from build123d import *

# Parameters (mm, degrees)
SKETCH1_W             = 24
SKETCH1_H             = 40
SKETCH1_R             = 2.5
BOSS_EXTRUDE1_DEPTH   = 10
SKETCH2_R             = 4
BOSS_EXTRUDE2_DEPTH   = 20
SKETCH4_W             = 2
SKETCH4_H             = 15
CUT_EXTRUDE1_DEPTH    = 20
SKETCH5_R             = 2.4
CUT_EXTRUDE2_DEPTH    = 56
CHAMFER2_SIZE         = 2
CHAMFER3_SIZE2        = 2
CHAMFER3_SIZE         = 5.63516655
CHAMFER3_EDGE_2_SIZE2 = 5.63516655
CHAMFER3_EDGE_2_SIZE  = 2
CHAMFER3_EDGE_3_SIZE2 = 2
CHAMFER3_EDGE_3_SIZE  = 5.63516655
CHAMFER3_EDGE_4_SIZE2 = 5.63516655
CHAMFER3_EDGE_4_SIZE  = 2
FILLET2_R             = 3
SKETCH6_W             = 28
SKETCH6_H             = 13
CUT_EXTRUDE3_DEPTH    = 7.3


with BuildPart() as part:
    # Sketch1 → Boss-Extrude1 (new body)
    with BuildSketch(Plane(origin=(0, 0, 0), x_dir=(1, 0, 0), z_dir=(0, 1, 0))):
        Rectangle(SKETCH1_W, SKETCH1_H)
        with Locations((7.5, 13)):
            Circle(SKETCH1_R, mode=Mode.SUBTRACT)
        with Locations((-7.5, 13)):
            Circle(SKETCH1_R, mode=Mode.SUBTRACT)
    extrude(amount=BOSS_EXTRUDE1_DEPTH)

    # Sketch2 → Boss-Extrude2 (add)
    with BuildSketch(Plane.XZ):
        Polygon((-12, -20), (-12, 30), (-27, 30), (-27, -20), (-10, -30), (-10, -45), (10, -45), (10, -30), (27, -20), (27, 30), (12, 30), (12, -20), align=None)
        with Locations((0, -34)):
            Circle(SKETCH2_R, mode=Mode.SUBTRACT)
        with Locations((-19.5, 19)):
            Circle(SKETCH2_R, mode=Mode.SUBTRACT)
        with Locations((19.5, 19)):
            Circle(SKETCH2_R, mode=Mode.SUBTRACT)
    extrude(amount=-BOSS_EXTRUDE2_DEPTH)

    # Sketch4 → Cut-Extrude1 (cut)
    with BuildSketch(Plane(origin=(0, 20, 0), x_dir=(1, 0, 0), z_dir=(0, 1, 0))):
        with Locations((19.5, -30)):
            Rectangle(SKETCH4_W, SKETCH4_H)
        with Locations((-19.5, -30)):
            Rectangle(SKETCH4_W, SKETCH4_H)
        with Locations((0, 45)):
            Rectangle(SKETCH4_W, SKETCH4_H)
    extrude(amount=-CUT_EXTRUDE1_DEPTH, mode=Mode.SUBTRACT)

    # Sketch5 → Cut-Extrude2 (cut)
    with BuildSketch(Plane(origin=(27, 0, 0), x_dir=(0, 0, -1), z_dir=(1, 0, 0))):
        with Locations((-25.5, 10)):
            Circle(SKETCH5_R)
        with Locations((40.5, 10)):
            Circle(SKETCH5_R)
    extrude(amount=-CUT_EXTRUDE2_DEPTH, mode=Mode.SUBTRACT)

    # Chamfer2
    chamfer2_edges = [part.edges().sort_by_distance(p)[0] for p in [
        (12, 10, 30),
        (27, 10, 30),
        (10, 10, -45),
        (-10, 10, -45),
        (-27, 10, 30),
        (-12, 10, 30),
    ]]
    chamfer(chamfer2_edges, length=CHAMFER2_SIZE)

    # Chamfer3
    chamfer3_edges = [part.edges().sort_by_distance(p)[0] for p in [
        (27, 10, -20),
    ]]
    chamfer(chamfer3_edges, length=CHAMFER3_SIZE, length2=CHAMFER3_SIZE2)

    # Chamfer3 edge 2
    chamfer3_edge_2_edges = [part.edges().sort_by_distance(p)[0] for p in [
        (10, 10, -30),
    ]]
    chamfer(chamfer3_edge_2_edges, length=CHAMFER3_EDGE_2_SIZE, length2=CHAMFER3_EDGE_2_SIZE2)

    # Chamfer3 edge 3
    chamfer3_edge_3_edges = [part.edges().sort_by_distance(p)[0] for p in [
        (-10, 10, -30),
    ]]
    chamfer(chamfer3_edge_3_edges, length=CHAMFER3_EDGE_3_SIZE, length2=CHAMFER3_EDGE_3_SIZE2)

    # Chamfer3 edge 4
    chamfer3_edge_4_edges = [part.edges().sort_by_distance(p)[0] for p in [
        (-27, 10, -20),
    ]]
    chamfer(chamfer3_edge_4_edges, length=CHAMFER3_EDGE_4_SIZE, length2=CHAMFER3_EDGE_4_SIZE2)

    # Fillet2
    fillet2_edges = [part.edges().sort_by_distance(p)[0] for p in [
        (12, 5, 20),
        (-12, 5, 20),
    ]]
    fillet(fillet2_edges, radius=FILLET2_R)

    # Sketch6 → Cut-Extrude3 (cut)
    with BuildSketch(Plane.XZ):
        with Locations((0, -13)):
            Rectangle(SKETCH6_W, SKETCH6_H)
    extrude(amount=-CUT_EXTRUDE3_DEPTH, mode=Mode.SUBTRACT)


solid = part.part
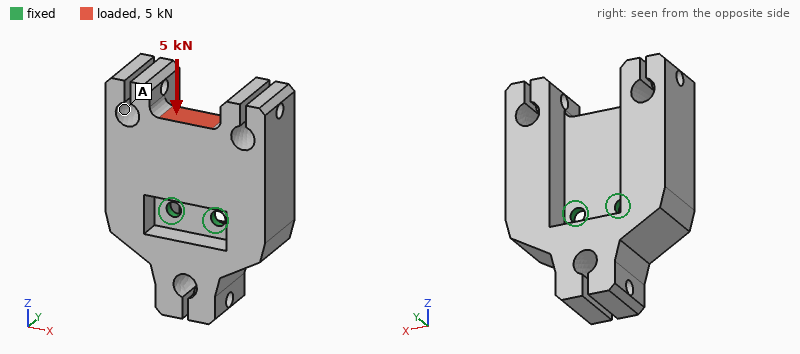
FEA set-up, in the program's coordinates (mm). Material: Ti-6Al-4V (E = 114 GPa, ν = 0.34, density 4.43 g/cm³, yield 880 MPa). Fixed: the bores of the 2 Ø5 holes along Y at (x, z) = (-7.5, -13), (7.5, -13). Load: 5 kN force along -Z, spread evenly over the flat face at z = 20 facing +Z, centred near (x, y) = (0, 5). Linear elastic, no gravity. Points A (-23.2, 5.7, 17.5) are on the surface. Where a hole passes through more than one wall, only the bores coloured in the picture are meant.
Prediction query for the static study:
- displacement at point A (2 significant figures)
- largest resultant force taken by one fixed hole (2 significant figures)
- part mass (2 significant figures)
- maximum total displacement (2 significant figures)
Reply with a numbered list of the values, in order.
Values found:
1. 0.091 mm
2. 2.6 kN
3. 200 g
4. 0.13 mm
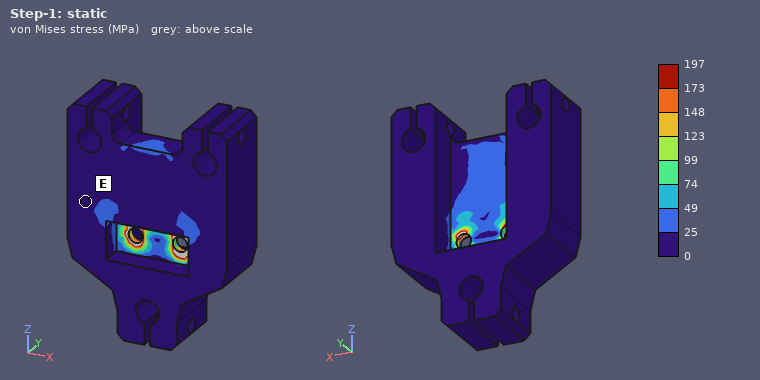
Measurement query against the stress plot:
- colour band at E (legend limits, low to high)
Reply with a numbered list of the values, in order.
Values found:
1. 0 to 25 MPa
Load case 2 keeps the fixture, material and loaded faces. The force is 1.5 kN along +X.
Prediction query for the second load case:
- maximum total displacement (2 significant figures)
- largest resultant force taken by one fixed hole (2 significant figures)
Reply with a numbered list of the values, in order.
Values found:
1. 28 µm
2. 2.8 kN
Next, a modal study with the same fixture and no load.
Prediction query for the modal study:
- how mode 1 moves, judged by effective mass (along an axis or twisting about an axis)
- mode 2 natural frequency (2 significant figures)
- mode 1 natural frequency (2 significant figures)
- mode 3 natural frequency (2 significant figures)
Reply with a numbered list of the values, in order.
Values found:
1. along Y
2. 3700 Hz
3. 1400 Hz
4. 4300 Hz
